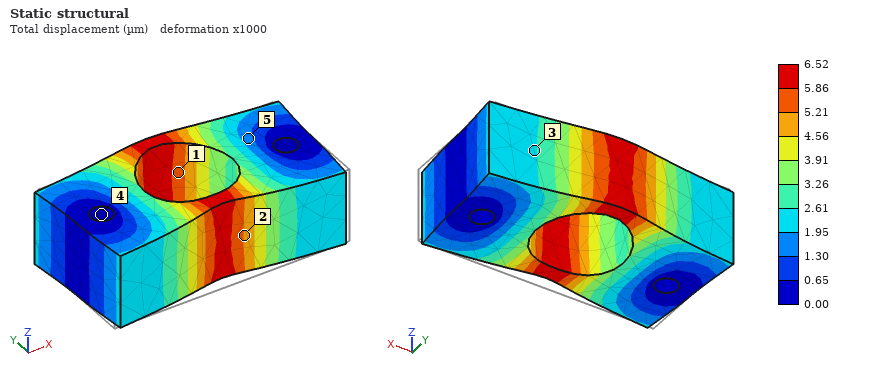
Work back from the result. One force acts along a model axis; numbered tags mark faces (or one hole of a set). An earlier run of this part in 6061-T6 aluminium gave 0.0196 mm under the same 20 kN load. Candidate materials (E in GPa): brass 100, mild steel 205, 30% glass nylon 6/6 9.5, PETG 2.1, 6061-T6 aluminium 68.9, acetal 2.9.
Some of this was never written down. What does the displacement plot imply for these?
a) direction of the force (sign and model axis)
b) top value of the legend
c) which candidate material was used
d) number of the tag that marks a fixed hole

+Y
6.52 µm
mild steel
4
